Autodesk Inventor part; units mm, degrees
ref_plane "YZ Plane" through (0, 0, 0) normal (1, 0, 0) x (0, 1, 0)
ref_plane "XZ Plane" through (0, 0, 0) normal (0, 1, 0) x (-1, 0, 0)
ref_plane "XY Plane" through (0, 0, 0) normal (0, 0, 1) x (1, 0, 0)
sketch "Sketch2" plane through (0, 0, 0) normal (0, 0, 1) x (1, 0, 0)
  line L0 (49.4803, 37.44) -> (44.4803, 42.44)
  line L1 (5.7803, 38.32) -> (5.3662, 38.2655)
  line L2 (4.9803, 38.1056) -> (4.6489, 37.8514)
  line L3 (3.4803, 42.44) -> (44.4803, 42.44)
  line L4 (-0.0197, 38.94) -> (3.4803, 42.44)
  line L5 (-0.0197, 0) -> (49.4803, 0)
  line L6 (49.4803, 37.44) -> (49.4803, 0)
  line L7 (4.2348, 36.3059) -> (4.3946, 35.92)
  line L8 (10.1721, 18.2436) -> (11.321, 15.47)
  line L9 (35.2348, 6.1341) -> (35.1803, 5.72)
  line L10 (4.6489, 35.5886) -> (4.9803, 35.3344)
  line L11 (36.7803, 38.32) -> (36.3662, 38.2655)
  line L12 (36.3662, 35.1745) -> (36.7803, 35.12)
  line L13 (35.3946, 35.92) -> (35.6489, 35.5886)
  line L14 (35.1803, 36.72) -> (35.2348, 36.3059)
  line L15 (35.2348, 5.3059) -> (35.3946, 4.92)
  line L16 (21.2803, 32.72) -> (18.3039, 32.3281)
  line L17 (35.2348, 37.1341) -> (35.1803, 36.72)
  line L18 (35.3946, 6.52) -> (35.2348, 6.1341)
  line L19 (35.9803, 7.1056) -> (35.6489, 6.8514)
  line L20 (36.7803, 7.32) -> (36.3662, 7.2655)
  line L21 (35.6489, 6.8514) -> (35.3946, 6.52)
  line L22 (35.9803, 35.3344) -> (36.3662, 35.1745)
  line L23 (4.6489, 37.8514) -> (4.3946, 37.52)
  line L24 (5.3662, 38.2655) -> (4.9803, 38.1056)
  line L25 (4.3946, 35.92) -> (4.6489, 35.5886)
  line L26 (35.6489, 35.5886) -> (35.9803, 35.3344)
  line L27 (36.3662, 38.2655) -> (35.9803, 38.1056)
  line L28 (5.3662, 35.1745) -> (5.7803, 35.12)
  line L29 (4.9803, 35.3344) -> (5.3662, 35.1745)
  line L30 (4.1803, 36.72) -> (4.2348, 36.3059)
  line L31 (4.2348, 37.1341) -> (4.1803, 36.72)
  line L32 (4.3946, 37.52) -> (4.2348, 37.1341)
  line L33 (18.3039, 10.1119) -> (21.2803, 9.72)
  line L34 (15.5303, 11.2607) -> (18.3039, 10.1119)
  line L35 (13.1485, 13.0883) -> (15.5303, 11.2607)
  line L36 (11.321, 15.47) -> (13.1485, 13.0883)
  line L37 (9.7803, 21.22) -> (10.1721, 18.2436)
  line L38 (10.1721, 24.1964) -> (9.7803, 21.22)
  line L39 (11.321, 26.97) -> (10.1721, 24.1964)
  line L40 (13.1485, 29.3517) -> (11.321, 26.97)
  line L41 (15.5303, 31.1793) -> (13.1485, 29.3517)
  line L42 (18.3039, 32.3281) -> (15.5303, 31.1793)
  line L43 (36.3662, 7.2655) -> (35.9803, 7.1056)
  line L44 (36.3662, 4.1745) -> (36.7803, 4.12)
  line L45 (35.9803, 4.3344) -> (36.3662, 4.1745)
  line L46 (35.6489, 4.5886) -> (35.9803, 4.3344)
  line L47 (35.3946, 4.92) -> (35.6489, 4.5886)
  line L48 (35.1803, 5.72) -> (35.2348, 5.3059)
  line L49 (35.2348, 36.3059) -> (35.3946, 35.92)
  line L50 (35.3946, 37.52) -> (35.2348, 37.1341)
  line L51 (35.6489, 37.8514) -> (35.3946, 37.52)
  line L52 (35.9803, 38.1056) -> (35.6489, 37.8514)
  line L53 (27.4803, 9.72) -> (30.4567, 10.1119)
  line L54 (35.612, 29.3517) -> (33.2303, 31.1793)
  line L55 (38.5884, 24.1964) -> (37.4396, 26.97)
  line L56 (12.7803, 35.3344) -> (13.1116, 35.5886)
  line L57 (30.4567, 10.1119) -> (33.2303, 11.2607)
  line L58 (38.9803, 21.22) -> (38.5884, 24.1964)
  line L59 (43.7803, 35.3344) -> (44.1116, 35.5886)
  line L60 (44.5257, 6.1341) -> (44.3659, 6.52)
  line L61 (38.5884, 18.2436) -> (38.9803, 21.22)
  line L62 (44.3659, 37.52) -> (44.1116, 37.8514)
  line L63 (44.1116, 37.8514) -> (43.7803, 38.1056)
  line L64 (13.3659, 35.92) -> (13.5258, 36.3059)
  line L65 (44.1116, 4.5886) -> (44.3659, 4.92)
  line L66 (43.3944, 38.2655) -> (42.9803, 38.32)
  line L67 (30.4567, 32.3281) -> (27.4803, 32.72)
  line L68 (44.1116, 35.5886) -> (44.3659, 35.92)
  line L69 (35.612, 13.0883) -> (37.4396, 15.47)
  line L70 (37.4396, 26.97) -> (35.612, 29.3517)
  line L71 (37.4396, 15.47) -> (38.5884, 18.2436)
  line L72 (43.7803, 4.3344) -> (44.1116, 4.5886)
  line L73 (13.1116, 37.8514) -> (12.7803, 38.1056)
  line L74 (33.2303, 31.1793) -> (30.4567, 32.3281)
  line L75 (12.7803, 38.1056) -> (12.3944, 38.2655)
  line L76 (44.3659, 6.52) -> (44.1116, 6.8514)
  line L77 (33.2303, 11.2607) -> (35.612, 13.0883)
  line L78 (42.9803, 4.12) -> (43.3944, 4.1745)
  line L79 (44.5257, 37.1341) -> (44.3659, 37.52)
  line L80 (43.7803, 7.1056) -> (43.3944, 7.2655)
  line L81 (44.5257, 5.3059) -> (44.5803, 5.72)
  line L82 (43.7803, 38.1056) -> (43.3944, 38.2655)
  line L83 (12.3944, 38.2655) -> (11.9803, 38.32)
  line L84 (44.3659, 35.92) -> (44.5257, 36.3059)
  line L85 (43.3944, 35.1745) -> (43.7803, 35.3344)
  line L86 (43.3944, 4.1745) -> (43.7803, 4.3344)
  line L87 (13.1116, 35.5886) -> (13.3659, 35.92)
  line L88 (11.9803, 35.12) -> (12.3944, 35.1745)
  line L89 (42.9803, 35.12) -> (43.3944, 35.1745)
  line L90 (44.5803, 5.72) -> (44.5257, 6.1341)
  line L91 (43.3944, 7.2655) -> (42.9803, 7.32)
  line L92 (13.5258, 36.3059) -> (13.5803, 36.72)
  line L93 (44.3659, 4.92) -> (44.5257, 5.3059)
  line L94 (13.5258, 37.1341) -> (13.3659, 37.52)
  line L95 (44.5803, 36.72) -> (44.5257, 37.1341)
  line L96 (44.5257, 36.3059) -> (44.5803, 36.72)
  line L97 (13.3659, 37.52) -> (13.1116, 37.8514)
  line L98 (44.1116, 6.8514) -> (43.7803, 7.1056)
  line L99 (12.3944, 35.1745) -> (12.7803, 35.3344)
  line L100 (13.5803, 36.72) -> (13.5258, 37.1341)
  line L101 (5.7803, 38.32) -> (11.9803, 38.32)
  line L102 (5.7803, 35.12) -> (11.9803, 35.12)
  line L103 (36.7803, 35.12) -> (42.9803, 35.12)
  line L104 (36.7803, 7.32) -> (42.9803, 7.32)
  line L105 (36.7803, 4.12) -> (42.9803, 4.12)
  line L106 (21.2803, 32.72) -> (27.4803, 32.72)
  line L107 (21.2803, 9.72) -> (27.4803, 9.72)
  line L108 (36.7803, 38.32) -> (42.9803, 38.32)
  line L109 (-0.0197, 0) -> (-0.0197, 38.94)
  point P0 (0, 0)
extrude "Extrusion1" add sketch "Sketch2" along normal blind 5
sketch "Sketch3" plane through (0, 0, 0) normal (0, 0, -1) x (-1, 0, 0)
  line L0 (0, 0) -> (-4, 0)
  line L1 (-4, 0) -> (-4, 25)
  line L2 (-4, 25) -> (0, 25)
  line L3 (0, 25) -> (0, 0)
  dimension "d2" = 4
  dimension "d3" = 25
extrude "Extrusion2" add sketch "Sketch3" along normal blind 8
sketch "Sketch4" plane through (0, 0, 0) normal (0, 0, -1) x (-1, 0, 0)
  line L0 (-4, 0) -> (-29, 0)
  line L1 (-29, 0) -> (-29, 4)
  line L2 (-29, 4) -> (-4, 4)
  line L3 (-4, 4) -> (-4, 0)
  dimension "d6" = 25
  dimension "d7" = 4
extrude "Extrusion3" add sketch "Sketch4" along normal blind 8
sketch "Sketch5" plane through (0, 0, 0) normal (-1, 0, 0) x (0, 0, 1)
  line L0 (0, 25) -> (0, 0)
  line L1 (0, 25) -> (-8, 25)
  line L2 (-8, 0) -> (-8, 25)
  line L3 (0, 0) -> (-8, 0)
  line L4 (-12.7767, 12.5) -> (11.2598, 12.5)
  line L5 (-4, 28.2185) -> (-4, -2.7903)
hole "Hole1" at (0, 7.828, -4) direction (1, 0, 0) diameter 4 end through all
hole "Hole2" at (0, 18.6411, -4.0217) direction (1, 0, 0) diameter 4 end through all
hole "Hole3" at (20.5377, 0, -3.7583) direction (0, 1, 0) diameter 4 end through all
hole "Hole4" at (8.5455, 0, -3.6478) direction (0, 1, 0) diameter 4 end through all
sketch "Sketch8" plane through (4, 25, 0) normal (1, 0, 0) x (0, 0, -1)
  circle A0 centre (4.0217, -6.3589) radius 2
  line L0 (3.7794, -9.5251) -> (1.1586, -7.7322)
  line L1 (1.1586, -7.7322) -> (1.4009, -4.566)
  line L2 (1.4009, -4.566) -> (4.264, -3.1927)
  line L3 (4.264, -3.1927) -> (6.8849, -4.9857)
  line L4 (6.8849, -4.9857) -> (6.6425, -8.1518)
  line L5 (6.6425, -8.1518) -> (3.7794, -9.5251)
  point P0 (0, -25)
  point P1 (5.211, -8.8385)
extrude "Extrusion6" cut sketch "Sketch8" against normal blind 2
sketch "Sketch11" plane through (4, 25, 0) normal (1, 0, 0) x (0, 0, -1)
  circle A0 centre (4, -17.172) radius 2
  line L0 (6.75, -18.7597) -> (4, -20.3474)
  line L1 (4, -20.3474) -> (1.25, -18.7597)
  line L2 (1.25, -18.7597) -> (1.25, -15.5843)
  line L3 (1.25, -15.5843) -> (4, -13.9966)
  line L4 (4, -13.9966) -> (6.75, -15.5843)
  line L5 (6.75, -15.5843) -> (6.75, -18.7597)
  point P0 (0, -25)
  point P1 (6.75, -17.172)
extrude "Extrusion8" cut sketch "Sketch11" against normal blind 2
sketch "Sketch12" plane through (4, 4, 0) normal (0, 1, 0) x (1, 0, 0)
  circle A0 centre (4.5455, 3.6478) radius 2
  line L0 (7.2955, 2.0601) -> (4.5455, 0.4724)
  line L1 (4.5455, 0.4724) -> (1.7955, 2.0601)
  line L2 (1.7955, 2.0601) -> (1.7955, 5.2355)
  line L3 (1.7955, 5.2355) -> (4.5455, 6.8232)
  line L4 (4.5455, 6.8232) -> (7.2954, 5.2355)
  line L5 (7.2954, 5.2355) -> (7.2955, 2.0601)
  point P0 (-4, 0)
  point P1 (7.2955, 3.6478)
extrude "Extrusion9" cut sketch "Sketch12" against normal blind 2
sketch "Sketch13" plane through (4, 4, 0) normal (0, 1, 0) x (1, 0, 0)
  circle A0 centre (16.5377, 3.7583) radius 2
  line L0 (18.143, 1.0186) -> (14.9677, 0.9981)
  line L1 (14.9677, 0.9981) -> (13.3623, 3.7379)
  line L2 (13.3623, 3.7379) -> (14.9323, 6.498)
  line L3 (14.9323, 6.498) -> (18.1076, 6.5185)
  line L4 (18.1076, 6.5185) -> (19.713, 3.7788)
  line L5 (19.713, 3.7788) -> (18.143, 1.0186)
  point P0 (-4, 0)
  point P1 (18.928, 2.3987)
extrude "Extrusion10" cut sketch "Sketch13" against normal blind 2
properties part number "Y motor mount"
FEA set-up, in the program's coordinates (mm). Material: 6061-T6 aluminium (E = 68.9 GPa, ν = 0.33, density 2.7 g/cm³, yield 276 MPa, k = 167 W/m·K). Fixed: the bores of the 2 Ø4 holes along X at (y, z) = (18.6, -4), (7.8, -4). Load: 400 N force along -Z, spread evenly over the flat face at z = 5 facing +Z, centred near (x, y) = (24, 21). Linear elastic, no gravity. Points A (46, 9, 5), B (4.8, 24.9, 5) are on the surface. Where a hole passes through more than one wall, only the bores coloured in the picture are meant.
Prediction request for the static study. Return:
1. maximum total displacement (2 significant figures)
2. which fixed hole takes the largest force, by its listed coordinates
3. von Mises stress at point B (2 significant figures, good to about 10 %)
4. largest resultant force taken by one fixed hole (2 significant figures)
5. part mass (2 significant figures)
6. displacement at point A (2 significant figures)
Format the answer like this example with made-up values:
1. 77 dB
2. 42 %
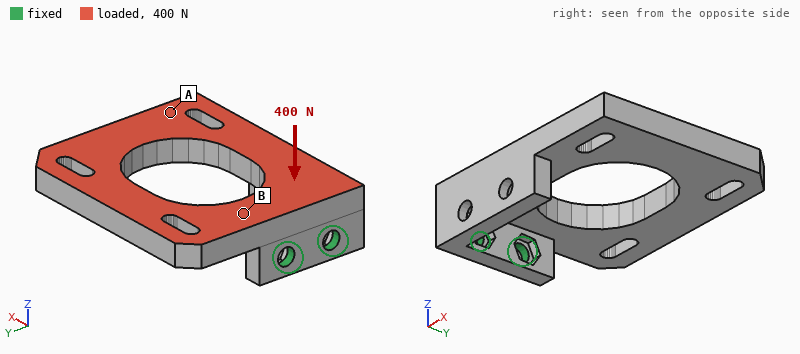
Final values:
1. 0.63 mm
2. (18.6, -4)
3. 61 MPa
4. 480 N
5. 23 g
6. 0.44 mm
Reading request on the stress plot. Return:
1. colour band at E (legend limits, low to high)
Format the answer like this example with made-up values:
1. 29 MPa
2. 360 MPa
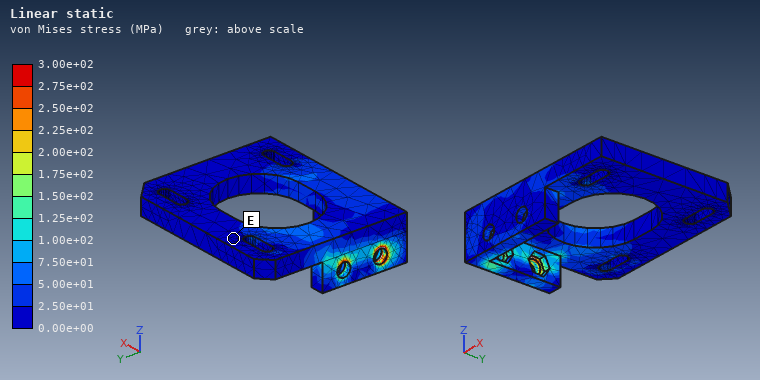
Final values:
1. 0.00e+00 to 2.50e+01 MPa
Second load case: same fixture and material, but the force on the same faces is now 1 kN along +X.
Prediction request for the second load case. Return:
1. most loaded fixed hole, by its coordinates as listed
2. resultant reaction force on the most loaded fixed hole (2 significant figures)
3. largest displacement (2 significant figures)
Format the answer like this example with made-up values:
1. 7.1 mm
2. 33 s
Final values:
1. (18.6, -4)
2. 1.0 kN
3. 0.38 mm
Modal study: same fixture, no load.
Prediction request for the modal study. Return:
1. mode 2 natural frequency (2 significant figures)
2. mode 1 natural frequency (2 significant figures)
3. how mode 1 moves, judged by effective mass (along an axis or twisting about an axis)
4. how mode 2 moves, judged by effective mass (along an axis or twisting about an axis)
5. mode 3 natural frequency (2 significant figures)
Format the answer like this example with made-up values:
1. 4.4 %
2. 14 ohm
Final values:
1. 2200 Hz
2. 1100 Hz
3. along Z
4. along Y
5. 3400 Hz
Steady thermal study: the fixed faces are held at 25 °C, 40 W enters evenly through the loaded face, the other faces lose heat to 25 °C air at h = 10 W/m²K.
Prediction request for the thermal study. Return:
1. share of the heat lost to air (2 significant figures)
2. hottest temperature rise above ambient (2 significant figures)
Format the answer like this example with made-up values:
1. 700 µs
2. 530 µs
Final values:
1. 3.9 %
2. 65 K
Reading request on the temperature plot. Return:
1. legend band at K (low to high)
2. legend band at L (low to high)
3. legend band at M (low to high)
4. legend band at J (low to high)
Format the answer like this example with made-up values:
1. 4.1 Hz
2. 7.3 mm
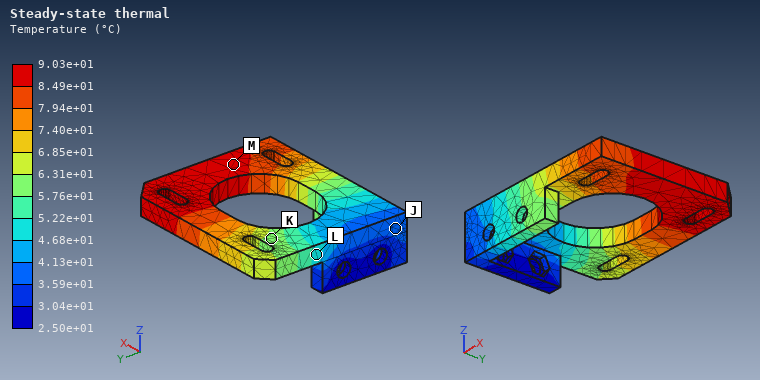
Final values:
1. 5.76e+01 to 6.31e+01 °C
2. 4.68e+01 to 5.22e+01 °C
3. 8.49e+01 to 9.03e+01 °C
4. 3.59e+01 to 4.13e+01 °C
